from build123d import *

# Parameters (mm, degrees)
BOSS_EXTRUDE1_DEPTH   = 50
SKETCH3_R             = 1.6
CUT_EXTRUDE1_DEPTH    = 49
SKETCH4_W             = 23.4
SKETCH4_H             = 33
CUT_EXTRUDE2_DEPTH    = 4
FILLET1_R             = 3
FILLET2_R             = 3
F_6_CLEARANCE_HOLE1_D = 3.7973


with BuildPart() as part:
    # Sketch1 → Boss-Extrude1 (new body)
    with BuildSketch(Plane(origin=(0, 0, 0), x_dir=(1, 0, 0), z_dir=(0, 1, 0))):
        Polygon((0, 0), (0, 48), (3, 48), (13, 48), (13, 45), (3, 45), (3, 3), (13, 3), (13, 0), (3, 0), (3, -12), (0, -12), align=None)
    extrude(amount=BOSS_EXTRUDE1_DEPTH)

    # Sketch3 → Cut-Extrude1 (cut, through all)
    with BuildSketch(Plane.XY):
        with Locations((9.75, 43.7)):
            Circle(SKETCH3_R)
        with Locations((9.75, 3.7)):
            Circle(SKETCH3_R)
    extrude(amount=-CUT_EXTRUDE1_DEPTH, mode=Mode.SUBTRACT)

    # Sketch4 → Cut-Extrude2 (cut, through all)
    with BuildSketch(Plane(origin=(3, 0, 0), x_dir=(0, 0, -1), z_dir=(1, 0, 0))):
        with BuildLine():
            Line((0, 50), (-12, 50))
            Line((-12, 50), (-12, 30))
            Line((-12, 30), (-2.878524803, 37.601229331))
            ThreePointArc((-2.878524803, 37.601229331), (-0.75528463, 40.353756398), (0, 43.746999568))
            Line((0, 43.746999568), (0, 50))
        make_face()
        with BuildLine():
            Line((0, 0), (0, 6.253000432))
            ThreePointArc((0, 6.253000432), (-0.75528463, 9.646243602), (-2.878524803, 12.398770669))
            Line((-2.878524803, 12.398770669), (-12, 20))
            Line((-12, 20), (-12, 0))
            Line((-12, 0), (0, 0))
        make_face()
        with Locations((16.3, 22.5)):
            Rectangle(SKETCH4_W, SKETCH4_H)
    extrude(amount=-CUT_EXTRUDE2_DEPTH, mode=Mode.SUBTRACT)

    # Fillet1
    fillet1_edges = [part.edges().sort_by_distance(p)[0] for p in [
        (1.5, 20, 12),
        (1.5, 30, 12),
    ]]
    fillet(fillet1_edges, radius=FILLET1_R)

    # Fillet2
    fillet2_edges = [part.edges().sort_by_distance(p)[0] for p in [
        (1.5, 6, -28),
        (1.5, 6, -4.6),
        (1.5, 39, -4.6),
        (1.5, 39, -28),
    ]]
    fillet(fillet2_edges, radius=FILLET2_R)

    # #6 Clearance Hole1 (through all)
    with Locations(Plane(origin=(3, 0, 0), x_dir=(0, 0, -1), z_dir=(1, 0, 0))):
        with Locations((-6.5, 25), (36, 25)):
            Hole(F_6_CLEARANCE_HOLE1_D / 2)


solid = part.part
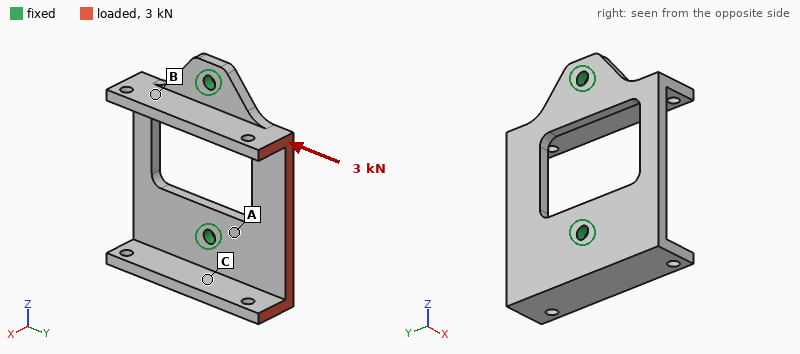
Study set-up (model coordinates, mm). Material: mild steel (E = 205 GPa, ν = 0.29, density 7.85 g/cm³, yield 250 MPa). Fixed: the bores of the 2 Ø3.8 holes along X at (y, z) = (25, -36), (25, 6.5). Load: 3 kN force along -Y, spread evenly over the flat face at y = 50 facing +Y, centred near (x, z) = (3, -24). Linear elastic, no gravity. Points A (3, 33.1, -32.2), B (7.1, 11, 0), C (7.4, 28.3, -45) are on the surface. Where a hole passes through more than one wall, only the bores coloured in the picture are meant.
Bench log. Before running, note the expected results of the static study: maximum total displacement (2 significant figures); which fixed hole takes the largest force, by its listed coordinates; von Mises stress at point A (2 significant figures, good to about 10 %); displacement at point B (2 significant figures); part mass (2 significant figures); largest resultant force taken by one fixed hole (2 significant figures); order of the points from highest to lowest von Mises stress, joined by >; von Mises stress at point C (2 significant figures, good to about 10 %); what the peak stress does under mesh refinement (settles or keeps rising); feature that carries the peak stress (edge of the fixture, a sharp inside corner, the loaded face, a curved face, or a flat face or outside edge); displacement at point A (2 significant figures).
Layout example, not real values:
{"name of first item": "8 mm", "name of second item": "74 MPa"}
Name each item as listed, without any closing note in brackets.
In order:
{"maximum total displacement": "40 µm", "which fixed hole takes the largest force, by its listed coordinates": "(25, -36)", "von Mises stress at point A": "66 MPa", "displacement at point B": "17 µm", "part mass": "67 g", "largest resultant force taken by one fixed hole": "2.0 kN", "order of the points from highest to lowest von Mises stress, joined by >": "A > C > B", "von Mises stress at point C": "23 MPa", "what the peak stress does under mesh refinement": "keeps rising", "feature that carries the peak stress": "edge of the fixture", "displacement at point A": "6.1 µm"}
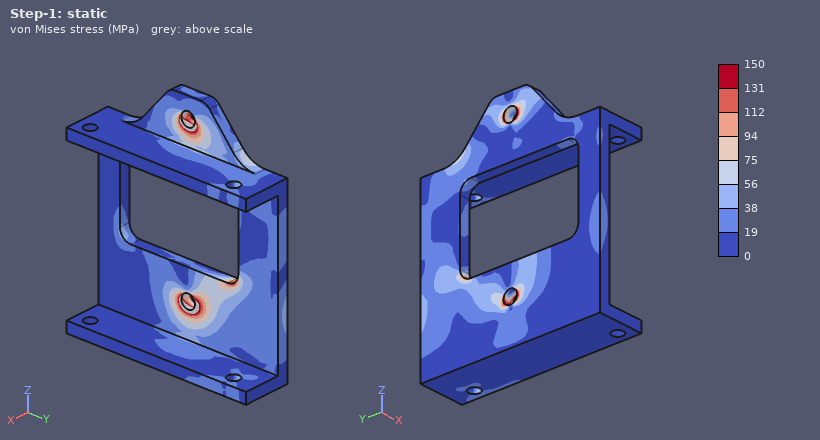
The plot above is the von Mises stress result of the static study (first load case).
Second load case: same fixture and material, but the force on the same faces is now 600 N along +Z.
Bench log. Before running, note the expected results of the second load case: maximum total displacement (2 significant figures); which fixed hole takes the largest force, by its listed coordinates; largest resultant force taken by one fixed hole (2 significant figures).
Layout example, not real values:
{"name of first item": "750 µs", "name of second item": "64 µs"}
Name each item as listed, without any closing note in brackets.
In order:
{"maximum total displacement": "20 µm", "which fixed hole takes the largest force, by its listed coordinates": "(25, -36)", "largest resultant force taken by one fixed hole": "430 N"}
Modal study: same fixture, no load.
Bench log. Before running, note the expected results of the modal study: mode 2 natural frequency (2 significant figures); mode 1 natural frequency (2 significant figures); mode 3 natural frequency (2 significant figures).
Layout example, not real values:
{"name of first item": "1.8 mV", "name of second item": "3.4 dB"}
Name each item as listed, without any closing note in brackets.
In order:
{"mode 2 natural frequency": "3900 Hz", "mode 1 natural frequency": "2900 Hz", "mode 3 natural frequency": "4800 Hz"}
